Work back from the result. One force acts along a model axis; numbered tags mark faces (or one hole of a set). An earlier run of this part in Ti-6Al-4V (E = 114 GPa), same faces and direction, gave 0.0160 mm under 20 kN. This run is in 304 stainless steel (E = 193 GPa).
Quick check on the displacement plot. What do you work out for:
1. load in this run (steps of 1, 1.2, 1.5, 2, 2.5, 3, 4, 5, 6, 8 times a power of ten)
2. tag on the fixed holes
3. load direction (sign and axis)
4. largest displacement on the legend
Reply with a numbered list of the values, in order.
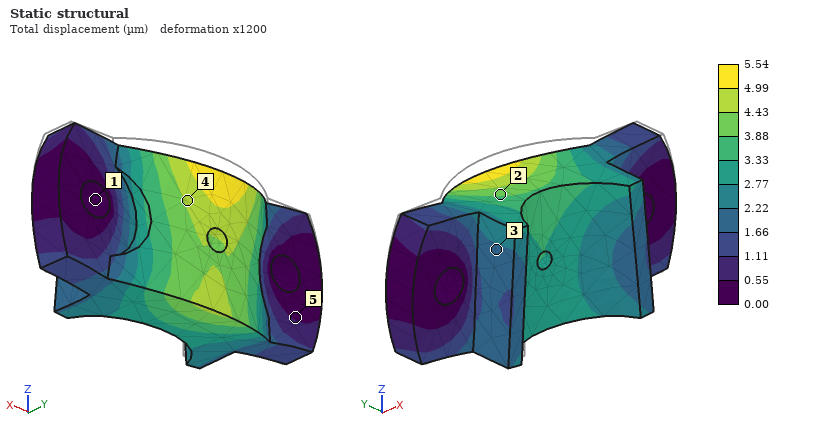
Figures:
1. 12 kN
2. 1
3. -Z
4. 5.54 µm
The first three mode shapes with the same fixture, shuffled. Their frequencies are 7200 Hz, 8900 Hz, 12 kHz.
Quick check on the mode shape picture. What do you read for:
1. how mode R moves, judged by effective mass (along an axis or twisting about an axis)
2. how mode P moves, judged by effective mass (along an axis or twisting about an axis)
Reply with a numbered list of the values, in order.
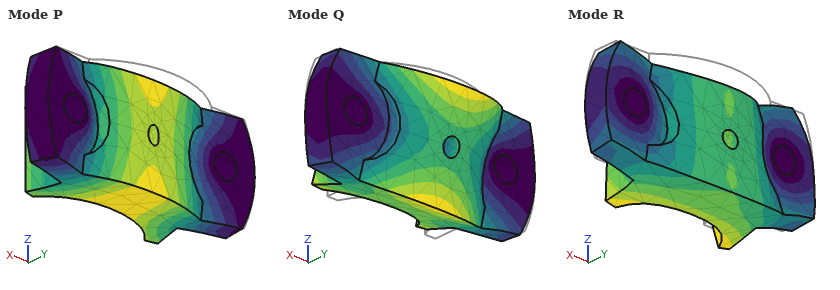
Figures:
1. along Z
2. along Y
